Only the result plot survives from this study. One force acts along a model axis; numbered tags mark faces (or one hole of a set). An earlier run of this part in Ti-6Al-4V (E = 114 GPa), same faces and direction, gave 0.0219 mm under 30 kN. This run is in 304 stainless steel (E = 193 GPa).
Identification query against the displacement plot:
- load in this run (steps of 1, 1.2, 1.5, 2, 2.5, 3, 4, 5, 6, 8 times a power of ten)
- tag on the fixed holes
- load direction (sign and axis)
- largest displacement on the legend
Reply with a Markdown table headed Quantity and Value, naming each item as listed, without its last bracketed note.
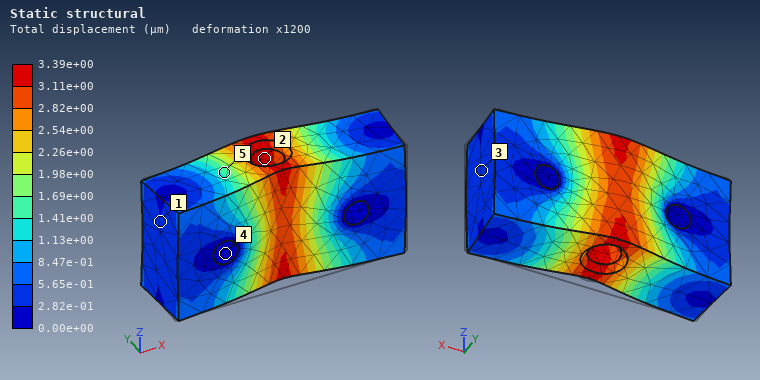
| Quantity | Value |
|---|---|
| load in this run | 8 kN |
| tag on the fixed holes | 4 |
| load direction | +Y |
| largest displacement on the legend | 3.39e+00 µm |
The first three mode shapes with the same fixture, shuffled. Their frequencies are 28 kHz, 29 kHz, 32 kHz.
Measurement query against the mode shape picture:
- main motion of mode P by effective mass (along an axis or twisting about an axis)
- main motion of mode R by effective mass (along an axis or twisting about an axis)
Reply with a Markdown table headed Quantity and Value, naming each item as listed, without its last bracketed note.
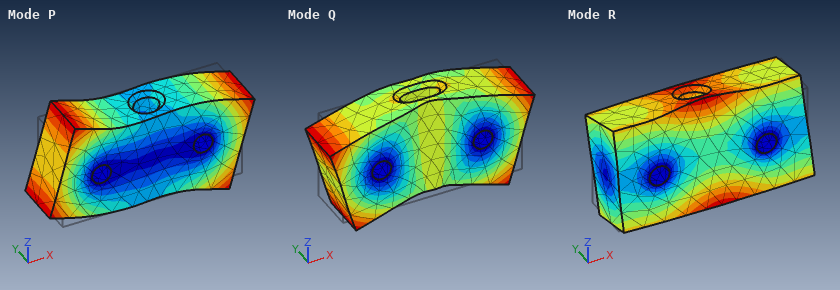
| Quantity | Value |
|---|---|
| main motion of mode P by effective mass | twisting about Y |
| main motion of mode R by effective mass | twisting about X |
